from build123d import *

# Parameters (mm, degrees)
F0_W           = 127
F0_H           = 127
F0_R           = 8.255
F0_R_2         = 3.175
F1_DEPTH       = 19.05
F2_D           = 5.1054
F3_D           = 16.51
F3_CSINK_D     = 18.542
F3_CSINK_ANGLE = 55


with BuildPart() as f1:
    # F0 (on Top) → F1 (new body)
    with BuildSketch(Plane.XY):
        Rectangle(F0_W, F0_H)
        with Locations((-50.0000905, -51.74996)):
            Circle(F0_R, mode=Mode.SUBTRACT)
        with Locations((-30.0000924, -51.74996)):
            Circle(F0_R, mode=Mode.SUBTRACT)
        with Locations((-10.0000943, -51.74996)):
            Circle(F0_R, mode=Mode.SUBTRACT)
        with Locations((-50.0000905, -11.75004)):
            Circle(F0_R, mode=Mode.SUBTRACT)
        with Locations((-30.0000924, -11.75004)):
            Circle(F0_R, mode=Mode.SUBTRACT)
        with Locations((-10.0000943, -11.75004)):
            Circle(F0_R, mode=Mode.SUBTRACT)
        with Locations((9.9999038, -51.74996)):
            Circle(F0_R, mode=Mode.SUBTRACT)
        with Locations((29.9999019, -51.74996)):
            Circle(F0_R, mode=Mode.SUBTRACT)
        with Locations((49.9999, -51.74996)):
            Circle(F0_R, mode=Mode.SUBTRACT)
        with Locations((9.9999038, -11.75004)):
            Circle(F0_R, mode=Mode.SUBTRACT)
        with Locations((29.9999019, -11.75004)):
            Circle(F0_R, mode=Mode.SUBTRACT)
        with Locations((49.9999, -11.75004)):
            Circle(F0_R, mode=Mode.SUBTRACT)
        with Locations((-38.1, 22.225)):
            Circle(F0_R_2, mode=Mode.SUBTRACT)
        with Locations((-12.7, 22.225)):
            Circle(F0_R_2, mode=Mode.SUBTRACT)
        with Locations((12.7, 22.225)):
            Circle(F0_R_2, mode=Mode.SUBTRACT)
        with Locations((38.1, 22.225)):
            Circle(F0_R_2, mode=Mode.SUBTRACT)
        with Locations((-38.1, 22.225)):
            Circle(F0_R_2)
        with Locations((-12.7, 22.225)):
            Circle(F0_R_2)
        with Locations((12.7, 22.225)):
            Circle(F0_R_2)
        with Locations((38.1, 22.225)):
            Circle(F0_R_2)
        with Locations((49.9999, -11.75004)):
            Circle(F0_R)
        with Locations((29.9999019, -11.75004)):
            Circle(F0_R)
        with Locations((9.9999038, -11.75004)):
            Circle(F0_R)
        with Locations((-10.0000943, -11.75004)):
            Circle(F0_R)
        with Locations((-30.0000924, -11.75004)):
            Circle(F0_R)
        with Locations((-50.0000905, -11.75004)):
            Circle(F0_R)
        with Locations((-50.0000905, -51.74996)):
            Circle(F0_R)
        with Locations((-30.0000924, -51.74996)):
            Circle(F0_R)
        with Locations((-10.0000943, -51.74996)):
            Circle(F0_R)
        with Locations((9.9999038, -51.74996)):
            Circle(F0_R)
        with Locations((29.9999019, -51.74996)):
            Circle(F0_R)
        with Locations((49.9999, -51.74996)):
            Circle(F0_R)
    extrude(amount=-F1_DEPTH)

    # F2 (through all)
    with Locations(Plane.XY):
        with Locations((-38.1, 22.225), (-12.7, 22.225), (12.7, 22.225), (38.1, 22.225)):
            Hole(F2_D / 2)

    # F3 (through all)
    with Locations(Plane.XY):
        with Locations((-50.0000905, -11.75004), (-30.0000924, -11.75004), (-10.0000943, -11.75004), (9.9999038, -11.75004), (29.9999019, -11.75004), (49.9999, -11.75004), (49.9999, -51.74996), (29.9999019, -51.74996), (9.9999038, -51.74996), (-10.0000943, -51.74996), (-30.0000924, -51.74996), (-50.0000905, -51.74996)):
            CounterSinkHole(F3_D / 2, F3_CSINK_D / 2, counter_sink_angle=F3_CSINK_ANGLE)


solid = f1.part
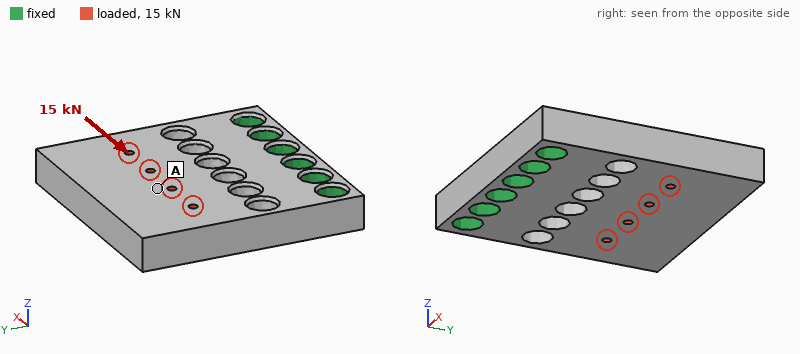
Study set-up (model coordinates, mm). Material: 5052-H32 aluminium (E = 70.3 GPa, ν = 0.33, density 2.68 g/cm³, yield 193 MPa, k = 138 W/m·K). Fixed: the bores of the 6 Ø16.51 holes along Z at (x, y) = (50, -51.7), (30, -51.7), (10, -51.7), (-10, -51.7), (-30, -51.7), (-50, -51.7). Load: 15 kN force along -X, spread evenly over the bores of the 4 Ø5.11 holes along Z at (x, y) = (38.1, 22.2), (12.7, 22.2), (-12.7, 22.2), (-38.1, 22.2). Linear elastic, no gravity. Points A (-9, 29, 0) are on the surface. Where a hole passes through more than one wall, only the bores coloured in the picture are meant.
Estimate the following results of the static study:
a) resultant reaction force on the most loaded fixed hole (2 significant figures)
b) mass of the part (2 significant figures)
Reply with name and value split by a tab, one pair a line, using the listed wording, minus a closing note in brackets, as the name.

resultant reaction force on the most loaded fixed hole	8.8 kN
mass of the part	690 g
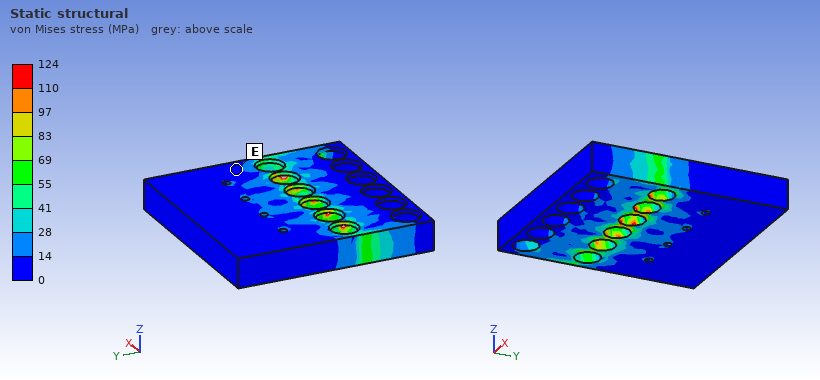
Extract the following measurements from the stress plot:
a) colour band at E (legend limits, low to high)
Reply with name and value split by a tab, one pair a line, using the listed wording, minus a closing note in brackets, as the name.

colour band at E	0 to 14 MPa
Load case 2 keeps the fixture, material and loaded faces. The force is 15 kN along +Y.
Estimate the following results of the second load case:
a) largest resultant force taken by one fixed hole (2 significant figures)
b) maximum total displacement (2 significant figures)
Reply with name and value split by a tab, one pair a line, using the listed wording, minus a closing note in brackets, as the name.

largest resultant force taken by one fixed hole	3.1 kN
maximum total displacement	14 µm
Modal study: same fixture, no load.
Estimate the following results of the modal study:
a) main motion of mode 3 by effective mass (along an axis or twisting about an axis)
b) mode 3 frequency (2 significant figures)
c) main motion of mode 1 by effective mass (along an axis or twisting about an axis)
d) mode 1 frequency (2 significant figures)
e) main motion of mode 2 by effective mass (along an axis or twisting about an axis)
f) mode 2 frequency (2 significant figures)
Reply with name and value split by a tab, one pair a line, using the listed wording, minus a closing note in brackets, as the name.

main motion of mode 3 by effective mass	along X
mode 3 frequency	3500 Hz
main motion of mode 1 by effective mass	along Z
mode 1 frequency	1000 Hz
main motion of mode 2 by effective mass	twisting about Y
mode 2 frequency	2300 Hz
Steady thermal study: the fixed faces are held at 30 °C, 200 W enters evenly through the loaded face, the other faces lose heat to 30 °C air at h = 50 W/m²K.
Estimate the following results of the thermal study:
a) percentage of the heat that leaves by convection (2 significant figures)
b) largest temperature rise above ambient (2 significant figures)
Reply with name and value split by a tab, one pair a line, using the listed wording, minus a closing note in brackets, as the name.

percentage of the heat that leaves by convection	30 %
largest temperature rise above ambient	54 K
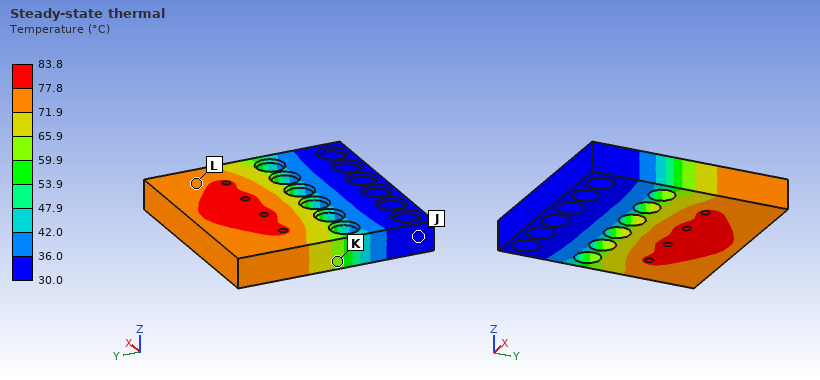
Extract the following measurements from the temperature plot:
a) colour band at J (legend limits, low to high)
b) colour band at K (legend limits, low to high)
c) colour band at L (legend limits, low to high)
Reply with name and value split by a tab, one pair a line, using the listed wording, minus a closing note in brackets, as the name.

colour band at J	30.0 to 36.0 °C
colour band at K	59.9 to 65.9 °C
colour band at L	71.9 to 77.8 °C
